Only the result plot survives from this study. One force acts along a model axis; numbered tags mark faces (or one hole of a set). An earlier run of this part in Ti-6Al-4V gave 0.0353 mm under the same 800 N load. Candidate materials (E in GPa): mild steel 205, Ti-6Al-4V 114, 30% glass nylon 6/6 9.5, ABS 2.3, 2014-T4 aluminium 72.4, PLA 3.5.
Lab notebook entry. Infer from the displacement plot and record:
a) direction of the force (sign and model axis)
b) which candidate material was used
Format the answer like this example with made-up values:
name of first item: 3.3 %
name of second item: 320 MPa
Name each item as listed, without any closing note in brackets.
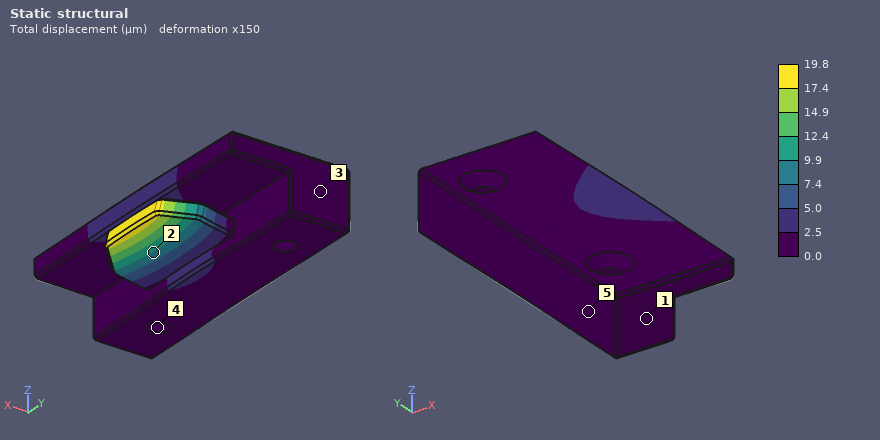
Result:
direction of the force: +Z
which candidate material was used: mild steel
